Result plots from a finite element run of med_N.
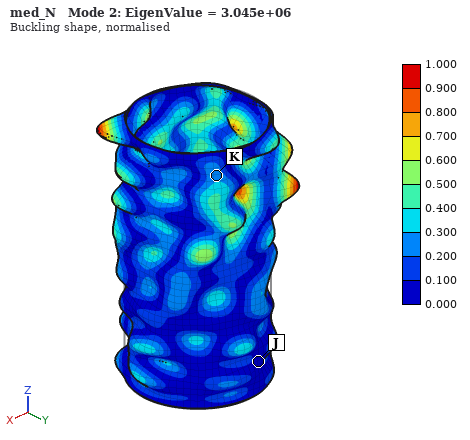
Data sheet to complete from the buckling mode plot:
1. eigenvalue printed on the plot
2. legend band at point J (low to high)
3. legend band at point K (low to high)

3.045e+06
0.000 to 0.100
0.200 to 0.300
